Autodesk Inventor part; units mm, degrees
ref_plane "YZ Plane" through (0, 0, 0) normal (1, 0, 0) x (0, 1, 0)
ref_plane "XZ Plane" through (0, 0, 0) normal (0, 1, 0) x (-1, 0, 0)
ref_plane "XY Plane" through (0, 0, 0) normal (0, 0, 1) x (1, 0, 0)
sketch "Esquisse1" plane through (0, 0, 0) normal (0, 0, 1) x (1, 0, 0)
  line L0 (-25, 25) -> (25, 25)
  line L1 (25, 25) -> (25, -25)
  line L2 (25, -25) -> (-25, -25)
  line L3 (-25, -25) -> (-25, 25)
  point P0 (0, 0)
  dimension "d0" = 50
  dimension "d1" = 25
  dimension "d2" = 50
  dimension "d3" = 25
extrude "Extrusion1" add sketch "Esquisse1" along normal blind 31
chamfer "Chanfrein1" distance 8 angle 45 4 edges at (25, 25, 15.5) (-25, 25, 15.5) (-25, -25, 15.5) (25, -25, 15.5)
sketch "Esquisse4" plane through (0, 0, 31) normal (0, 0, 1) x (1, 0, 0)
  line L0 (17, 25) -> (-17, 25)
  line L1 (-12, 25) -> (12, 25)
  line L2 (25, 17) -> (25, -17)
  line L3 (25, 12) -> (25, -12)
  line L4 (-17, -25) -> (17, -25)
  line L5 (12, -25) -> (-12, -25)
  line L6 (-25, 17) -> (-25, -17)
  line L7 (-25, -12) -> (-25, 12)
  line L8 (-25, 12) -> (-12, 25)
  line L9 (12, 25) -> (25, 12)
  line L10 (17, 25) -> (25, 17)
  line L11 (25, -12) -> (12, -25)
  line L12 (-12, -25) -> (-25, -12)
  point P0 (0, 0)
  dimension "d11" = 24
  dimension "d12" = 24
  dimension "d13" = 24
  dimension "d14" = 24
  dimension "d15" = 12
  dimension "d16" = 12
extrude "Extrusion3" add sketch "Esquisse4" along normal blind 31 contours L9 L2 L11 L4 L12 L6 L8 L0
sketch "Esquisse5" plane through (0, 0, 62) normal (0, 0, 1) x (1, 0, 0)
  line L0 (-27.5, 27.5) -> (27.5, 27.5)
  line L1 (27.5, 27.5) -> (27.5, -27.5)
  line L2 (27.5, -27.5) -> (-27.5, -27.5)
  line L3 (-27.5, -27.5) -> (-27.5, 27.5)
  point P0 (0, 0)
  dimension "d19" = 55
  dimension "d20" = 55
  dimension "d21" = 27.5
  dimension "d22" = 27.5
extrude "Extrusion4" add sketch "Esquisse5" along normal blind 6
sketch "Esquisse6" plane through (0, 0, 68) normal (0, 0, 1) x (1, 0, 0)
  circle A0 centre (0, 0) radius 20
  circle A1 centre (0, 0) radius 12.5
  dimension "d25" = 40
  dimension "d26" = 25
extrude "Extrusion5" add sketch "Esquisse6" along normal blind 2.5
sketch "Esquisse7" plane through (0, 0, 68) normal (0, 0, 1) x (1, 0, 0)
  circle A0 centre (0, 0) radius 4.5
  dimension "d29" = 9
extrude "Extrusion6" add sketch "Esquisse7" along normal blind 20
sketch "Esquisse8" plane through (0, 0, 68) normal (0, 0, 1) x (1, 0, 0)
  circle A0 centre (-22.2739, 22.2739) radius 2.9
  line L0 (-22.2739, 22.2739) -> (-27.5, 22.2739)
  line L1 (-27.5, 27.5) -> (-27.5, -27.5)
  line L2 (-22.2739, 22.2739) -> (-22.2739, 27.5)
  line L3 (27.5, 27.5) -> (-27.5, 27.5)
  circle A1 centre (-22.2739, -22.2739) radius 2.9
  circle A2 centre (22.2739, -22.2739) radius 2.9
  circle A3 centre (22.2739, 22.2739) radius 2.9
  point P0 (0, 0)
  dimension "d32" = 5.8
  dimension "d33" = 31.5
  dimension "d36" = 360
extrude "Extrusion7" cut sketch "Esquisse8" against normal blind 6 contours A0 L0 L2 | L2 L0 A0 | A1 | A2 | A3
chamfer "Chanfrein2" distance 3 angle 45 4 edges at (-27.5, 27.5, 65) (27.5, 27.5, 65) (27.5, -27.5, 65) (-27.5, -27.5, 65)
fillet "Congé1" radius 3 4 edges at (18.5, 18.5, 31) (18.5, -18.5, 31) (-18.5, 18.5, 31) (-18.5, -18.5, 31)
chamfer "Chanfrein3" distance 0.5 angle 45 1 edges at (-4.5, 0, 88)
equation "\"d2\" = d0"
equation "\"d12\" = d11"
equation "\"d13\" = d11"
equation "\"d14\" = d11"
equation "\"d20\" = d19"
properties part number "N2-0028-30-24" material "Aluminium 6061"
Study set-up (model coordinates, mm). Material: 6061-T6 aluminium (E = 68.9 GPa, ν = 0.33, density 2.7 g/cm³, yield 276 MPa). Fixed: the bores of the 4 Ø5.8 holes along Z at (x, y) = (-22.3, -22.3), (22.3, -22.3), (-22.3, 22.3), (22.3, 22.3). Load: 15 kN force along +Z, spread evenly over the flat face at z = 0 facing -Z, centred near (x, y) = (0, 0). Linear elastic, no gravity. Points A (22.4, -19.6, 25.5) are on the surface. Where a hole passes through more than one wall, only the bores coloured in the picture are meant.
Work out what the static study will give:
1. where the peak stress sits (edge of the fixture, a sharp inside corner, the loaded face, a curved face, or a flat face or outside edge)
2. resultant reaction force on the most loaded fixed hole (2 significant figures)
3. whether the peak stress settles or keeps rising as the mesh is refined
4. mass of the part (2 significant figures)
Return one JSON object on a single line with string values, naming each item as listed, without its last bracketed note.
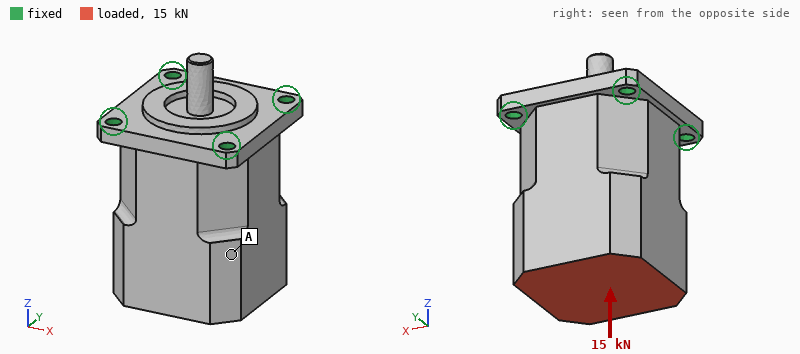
{"where the peak stress sits": "edge of the fixture", "resultant reaction force on the most loaded fixed hole": "4.0 kN", "whether the peak stress settles or keeps rising as the mesh is refined": "keeps rising", "mass of the part": "440 g"}
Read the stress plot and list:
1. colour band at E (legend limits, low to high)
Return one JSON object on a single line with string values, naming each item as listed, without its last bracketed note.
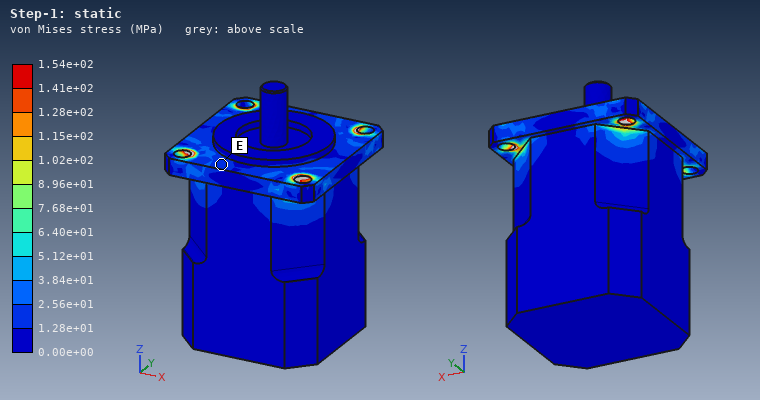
{"colour band at E": "1.28e+01 to 2.56e+01 MPa"}
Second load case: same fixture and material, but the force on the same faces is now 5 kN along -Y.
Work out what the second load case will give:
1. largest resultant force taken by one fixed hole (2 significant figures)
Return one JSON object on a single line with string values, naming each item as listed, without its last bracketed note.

{"largest resultant force taken by one fixed hole": "4.4 kN"}
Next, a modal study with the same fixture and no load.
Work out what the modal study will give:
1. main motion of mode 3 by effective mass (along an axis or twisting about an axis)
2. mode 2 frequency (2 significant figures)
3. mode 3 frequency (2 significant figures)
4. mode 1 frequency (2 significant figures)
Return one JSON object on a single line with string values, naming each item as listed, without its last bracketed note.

{"main motion of mode 3 by effective mass": "along Z", "mode 2 frequency": "3300 Hz", "mode 3 frequency": "6800 Hz", "mode 1 frequency": "3300 Hz"}
